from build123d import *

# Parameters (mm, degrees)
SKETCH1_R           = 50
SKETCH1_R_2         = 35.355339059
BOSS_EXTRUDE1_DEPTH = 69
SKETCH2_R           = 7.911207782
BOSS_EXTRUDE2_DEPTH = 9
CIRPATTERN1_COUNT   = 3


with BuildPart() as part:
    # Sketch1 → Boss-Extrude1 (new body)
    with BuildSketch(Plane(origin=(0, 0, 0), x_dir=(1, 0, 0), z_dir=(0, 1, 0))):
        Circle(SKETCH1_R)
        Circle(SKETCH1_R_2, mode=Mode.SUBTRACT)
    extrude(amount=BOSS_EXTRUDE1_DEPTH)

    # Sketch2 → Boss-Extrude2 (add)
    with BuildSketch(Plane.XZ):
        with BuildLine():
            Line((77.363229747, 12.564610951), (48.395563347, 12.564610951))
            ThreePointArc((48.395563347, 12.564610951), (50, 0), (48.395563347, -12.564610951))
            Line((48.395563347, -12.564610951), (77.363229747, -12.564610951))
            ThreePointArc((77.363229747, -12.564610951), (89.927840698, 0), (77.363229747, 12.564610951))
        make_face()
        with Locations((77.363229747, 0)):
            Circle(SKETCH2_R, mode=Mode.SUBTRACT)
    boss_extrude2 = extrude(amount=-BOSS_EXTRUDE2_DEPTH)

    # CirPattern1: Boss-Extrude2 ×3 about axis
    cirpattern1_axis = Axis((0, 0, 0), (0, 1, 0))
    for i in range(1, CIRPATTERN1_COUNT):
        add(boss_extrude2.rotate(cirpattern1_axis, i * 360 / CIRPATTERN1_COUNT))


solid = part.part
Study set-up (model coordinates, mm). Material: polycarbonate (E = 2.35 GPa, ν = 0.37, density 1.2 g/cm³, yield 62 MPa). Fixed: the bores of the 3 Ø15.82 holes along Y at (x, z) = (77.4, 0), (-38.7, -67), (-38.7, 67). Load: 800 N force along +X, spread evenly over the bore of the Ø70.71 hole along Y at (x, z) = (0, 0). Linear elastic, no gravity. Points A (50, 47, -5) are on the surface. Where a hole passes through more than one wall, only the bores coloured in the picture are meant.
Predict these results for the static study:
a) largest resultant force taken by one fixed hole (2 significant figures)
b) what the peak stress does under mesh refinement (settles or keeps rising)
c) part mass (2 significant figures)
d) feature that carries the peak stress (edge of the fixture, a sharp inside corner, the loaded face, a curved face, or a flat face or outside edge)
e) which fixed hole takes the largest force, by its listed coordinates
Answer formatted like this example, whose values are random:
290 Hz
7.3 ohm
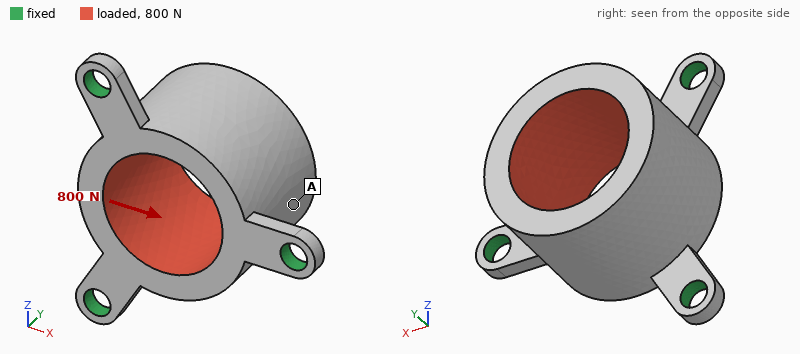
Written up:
440 N
keeps rising
350 g
edge of the fixture
(77.4, 0)
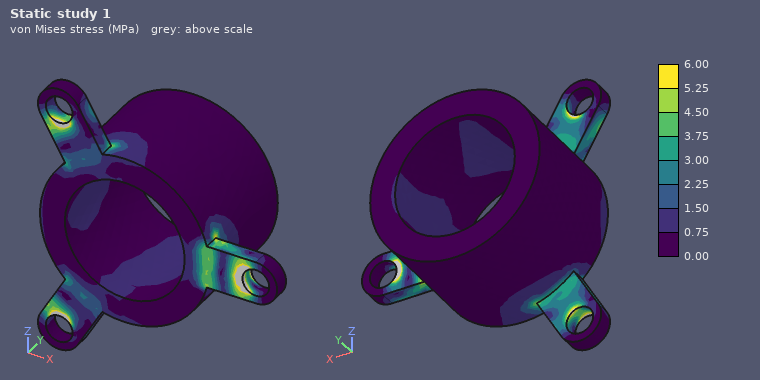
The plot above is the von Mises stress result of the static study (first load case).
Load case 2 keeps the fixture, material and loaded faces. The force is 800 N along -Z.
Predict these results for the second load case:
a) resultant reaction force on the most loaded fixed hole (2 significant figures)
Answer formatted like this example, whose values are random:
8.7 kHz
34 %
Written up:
390 N
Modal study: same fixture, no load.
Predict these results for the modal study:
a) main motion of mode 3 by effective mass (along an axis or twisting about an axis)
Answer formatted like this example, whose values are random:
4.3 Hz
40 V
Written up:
along Y
